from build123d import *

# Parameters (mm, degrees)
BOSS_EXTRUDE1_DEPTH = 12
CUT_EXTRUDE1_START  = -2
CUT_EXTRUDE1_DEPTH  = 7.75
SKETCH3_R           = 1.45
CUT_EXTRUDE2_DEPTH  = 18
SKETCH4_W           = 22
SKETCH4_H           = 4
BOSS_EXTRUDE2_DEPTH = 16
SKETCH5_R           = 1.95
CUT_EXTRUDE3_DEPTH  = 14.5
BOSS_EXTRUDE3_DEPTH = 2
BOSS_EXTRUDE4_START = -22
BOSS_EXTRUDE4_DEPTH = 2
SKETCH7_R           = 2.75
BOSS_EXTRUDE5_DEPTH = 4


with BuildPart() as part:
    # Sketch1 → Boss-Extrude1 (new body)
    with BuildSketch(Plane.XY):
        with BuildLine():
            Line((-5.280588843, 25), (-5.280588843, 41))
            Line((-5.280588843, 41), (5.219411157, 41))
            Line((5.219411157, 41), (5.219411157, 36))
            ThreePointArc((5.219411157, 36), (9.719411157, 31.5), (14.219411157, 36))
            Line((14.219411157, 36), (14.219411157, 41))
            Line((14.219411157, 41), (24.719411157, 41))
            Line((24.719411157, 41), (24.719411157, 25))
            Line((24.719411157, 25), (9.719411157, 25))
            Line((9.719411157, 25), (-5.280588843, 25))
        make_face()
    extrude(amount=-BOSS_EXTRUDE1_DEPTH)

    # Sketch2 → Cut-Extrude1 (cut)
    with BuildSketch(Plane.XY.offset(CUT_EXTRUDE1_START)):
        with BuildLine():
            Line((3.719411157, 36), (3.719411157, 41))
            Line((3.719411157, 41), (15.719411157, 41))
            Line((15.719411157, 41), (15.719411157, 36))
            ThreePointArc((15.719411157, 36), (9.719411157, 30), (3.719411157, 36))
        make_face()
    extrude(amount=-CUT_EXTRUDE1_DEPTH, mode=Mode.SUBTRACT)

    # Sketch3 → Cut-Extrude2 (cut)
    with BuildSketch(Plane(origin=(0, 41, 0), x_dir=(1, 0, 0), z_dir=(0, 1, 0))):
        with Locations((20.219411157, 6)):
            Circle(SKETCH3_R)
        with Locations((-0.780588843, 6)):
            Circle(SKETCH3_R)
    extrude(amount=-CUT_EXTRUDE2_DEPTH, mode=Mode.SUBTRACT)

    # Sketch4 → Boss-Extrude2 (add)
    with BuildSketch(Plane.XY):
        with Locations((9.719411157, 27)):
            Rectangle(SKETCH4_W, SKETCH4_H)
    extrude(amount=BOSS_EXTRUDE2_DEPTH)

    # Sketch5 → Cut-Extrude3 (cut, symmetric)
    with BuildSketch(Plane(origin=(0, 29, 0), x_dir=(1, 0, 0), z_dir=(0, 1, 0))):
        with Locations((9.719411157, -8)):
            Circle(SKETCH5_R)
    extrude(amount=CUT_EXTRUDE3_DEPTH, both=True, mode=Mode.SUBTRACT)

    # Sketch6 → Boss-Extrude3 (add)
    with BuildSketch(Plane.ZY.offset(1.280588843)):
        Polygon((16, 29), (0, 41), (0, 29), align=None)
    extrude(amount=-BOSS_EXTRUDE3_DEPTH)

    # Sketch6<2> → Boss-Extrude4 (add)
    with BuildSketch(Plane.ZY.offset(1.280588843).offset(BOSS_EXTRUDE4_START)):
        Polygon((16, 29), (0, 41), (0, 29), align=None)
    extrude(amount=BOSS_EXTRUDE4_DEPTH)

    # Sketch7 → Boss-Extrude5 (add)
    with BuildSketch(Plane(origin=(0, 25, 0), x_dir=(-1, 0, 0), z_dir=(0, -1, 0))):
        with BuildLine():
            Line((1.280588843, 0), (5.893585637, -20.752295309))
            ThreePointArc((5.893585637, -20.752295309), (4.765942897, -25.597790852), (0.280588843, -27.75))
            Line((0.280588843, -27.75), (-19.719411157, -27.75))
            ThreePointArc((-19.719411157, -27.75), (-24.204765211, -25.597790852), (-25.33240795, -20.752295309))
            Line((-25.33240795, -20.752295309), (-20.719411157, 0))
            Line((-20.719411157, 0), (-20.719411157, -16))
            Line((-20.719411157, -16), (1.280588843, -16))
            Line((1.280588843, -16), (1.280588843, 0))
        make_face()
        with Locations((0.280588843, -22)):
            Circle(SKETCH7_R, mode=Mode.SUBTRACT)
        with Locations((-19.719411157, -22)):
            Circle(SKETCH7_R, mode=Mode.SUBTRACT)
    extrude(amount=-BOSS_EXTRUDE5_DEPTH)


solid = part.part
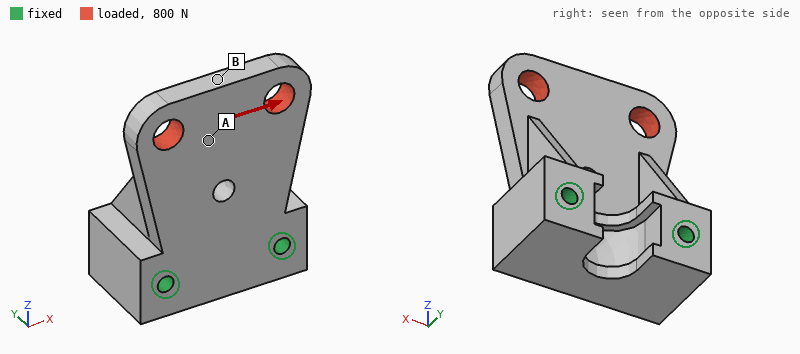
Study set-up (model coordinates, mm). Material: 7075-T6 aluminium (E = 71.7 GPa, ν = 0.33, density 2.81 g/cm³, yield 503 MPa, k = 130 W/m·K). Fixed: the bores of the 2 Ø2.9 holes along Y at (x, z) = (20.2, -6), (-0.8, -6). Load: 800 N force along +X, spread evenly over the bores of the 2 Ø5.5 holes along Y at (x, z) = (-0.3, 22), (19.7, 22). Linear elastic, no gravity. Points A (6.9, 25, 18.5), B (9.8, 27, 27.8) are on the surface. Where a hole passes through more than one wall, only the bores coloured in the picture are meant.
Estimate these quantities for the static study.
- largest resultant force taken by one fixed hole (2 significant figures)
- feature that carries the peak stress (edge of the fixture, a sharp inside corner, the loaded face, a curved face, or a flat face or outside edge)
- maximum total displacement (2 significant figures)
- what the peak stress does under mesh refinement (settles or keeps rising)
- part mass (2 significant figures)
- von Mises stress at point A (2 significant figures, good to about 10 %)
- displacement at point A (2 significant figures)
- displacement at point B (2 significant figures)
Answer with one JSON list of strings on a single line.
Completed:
["1.1 kN", "a sharp inside corner", "32 µm", "keeps rising", "21 g", "11 MPa", "16 µm", "26 µm"]
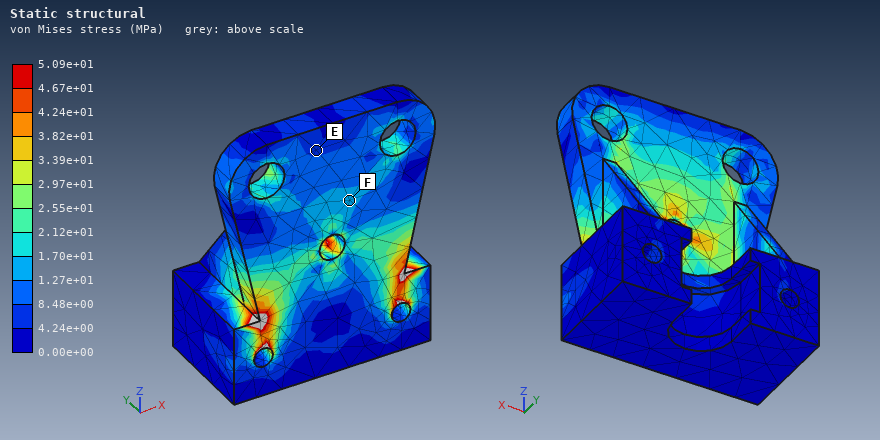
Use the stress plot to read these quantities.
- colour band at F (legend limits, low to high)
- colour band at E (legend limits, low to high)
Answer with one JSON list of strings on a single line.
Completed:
["1.27e+01 to 1.70e+01 MPa", "4.24e+00 to 8.48e+00 MPa"]
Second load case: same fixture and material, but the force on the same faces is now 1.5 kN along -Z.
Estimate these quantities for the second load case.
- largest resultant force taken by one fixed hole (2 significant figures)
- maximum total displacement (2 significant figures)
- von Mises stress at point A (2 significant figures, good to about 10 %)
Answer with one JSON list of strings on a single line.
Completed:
["760 N", "18 µm", "10 MPa"]
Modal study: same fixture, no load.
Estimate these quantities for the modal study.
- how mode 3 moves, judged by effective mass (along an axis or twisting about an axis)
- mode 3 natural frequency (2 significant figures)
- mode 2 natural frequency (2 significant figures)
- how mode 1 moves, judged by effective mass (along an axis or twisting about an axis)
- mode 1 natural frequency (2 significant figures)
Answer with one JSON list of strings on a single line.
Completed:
["along X", "16 kHz", "11 kHz", "along Y", "7000 Hz"]
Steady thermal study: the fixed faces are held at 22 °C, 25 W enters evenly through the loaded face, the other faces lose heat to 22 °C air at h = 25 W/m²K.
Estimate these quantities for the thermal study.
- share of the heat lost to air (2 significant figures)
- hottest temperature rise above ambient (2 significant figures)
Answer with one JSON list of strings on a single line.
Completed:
["5.8 %", "48 K"]
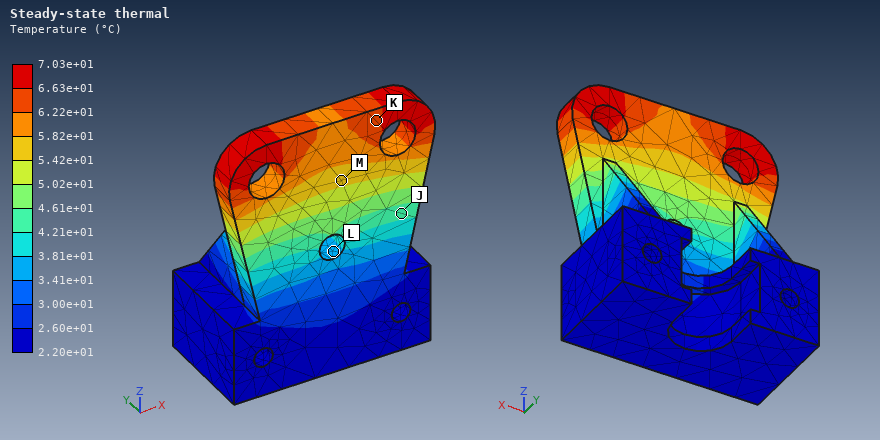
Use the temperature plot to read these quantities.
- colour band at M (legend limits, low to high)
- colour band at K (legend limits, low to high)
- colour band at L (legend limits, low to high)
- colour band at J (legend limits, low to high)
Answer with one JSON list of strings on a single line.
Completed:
["5.42e+01 to 5.82e+01 °C", "6.22e+01 to 6.63e+01 °C", "3.41e+01 to 3.81e+01 °C", "4.21e+01 to 4.61e+01 °C"]
